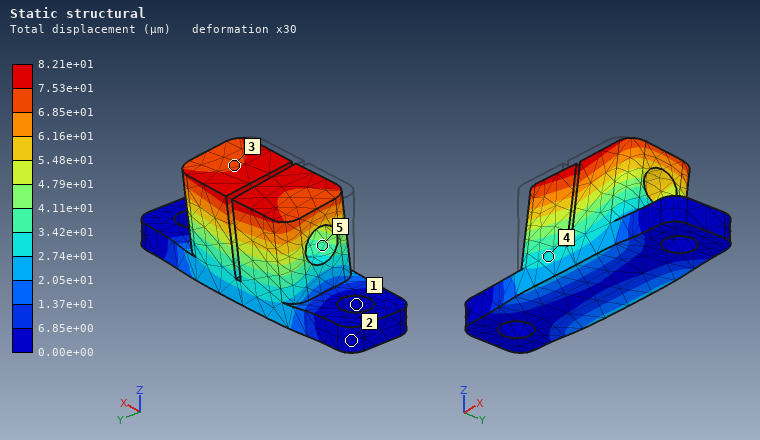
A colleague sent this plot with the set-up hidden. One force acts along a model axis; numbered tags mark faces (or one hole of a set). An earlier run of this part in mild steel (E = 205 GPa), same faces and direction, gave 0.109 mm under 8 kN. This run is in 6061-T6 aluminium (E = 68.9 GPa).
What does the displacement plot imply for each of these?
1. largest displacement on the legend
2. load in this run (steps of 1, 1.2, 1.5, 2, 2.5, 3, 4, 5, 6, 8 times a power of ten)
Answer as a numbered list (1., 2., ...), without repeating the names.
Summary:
1. 8.21e+01 µm
2. 2 kN
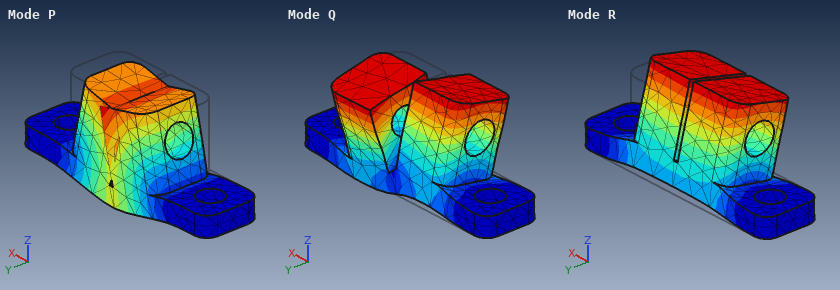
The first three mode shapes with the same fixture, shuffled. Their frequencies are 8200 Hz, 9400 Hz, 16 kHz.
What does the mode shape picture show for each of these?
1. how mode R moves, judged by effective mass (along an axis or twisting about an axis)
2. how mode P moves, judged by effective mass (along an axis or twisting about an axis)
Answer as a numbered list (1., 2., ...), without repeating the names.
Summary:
1. along Y
2. along Z
